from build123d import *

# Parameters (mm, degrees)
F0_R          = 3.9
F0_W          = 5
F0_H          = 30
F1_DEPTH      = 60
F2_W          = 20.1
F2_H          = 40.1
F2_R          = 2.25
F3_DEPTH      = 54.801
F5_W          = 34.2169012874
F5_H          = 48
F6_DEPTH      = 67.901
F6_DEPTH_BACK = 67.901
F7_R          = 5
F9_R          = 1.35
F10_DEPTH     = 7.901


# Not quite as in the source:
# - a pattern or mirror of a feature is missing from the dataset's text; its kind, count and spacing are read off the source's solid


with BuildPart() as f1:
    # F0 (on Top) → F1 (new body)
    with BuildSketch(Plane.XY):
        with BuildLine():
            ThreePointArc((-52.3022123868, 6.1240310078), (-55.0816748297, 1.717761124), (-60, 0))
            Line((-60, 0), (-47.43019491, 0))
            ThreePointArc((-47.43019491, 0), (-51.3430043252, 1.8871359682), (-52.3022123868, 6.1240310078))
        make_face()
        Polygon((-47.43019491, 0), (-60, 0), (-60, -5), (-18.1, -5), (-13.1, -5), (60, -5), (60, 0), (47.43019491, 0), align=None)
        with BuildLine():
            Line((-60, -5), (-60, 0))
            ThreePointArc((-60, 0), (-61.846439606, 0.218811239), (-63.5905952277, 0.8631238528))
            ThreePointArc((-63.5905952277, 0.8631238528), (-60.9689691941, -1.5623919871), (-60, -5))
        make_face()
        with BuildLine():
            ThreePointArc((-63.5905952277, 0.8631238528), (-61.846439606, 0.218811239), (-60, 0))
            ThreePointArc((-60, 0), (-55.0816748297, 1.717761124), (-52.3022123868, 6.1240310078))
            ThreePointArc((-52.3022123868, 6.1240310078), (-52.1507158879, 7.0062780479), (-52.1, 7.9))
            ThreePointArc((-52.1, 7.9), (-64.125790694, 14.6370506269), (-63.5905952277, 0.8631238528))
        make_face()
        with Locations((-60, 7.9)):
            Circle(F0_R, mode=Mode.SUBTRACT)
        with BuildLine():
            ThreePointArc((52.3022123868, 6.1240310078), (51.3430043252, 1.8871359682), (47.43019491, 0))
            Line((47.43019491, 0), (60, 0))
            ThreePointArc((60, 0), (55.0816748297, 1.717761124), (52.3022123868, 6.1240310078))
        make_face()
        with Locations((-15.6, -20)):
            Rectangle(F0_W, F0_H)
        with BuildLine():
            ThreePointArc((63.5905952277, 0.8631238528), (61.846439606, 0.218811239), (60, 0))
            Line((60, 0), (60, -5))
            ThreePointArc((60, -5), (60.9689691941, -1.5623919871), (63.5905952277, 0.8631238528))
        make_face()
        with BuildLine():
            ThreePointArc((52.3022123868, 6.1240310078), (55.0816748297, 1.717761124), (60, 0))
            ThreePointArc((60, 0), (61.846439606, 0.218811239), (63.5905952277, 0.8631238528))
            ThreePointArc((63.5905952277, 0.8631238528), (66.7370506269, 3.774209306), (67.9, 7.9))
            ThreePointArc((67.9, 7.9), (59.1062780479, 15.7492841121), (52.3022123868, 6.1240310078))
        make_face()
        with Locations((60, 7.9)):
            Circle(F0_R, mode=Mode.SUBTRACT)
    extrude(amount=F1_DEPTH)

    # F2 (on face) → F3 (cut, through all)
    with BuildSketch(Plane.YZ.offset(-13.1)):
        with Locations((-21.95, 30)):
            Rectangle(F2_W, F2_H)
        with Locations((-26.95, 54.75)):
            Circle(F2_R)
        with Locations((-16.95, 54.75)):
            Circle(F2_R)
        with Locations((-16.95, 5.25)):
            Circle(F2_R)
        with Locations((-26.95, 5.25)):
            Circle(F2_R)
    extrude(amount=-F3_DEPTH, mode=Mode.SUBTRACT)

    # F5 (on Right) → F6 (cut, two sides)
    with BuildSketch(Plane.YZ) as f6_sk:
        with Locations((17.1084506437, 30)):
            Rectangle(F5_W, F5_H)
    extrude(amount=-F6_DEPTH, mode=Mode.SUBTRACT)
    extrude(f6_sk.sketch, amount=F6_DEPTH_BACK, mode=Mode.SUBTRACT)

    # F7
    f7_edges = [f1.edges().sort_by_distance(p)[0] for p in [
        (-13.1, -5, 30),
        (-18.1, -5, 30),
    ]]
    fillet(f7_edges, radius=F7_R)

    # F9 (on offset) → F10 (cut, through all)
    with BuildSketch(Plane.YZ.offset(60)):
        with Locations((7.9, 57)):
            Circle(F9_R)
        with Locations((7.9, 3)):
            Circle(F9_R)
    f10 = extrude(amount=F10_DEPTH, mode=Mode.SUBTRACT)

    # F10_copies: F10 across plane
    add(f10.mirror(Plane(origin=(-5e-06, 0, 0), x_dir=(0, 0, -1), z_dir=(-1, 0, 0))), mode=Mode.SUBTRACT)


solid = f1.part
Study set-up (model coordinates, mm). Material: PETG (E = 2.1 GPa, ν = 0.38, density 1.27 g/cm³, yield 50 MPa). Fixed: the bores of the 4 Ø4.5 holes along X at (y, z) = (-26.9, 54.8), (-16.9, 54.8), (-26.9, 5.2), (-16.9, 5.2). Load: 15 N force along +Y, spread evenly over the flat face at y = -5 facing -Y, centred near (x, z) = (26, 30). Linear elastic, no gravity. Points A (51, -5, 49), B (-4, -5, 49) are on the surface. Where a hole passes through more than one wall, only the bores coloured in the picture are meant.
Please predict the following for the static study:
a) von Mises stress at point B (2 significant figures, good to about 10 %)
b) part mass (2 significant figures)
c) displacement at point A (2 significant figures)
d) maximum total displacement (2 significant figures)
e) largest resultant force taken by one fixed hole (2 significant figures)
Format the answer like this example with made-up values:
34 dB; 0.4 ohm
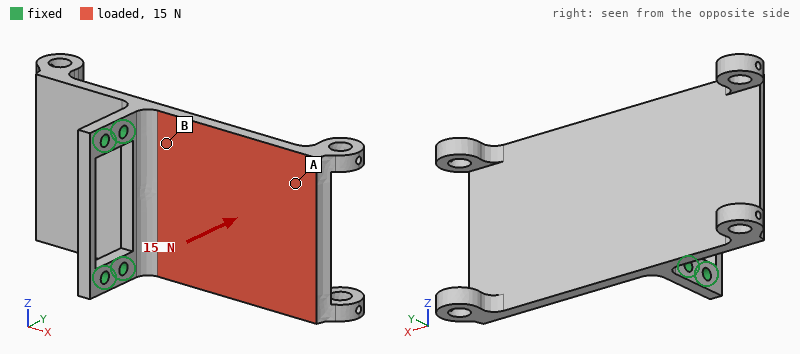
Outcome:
1.7 MPa; 58 g; 1.3 mm; 1.7 mm; 10 N
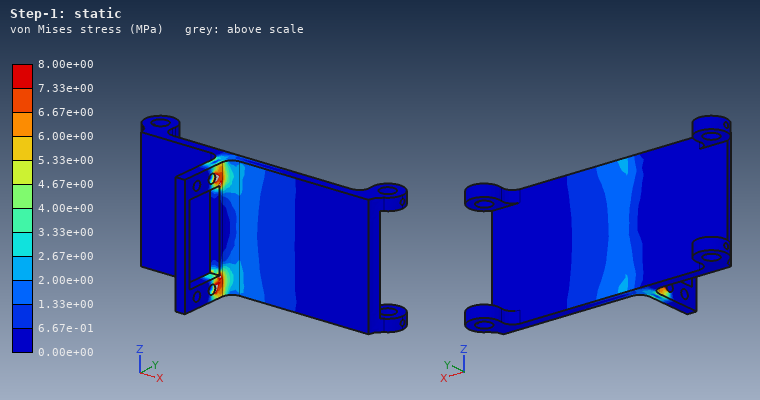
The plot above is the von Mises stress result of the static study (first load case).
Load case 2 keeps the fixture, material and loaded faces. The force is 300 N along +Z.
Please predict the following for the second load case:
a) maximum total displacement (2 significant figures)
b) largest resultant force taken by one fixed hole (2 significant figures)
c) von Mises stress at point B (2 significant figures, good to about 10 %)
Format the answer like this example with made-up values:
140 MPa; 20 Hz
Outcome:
1.4 mm; 310 N; 7.5 MPa
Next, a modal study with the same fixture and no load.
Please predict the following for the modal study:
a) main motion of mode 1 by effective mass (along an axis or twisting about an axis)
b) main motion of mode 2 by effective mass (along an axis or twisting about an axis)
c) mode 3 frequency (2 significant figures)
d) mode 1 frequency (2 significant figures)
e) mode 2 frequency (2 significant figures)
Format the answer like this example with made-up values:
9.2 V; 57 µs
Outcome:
along Y; along Y; 380 Hz; 100 Hz; 320 Hz
